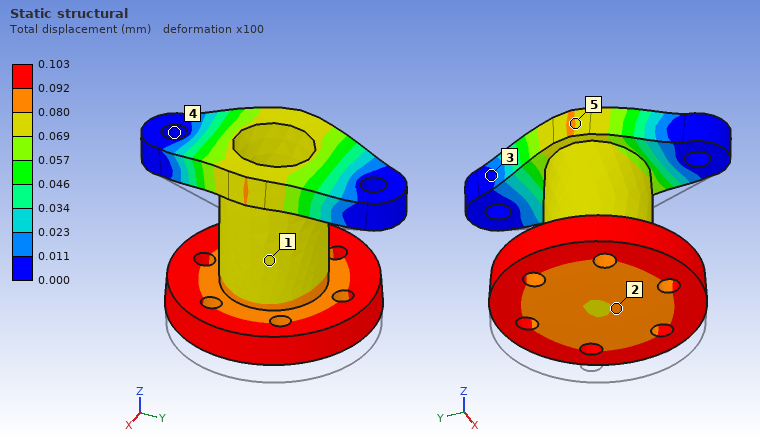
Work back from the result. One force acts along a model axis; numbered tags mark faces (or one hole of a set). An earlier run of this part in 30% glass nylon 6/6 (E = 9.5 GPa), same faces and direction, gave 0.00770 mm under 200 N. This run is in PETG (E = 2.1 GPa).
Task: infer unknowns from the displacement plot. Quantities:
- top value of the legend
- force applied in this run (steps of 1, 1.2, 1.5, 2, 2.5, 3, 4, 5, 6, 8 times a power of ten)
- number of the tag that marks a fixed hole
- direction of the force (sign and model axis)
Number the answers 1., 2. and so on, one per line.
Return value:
1. 0.103 mm
2. 600 N
3. 4
4. +Z
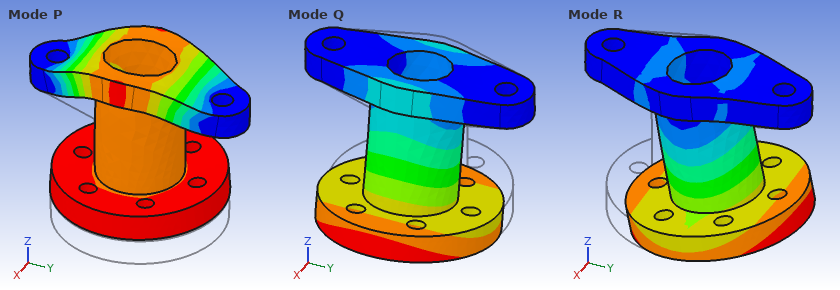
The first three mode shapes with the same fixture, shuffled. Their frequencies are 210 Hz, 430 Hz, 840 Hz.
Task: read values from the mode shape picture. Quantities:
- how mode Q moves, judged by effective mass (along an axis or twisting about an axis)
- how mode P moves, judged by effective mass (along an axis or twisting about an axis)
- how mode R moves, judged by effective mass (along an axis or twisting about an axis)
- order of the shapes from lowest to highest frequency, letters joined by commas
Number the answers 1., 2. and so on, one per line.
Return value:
1. along X
2. along Z
3. along Y
4. Q, R, P
